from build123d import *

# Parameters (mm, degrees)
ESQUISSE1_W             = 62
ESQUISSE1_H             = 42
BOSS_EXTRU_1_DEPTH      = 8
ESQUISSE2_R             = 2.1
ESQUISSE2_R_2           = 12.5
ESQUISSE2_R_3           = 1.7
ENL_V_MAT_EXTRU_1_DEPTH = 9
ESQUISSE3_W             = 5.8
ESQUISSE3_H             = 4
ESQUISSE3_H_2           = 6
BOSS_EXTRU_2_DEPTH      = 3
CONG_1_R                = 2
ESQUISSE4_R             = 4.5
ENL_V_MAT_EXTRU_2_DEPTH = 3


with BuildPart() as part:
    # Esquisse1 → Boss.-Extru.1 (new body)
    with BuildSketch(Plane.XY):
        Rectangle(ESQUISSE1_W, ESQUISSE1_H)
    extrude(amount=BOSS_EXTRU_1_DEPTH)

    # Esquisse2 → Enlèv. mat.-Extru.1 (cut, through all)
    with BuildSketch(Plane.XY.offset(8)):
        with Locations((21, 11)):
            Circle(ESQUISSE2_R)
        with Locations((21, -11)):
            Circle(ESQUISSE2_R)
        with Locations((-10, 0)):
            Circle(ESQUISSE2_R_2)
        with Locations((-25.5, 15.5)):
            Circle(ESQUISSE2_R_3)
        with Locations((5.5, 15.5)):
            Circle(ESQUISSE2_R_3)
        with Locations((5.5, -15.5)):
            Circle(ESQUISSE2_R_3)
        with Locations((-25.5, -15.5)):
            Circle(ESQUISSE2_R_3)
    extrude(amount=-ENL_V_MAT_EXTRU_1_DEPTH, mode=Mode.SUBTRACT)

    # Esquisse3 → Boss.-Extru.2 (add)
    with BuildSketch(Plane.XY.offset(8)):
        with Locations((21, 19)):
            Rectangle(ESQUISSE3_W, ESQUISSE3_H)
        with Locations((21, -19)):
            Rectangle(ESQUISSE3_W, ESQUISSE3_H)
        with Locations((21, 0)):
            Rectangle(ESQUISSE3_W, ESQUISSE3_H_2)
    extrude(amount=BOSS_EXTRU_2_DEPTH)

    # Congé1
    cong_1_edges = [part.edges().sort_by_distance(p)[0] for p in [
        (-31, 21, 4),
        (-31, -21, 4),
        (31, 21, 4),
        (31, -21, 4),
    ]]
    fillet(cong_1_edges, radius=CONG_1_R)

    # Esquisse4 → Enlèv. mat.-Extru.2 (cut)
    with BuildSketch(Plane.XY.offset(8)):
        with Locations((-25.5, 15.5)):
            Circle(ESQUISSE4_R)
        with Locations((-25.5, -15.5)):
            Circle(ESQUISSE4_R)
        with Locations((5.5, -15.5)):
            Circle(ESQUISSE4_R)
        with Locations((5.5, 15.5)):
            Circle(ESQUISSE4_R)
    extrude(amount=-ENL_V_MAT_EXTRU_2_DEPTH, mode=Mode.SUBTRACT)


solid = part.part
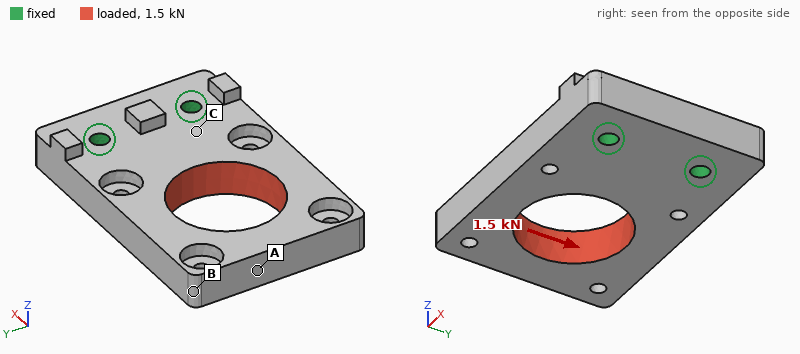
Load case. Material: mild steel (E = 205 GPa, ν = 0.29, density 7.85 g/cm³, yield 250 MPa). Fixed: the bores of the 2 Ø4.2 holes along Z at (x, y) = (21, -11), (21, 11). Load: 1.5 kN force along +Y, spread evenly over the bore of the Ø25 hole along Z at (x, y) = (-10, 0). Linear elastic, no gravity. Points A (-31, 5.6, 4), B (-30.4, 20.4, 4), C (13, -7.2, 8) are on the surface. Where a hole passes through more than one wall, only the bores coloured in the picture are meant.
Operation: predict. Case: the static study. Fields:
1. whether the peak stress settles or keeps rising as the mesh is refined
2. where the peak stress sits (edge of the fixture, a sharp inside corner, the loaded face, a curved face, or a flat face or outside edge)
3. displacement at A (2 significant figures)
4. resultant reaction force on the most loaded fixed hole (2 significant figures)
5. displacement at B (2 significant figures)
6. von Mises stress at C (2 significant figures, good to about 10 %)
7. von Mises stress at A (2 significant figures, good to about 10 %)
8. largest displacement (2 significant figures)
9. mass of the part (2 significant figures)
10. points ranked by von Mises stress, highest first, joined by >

keeps rising
a sharp inside corner
14 µm
2.0 kN
15 µm
16 MPa
10 MPa
16 µm
130 g
C > A > B
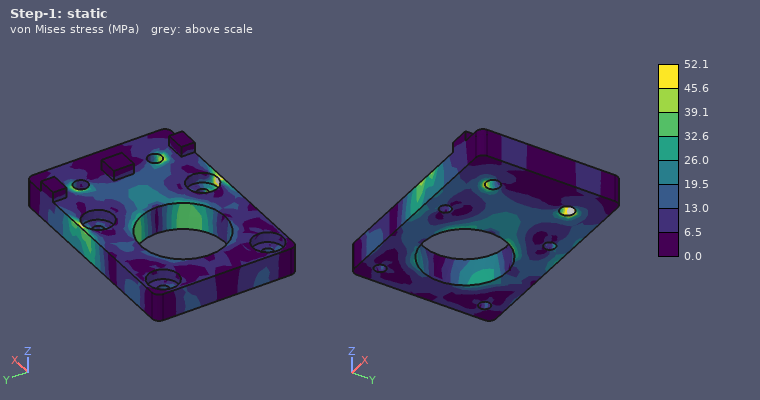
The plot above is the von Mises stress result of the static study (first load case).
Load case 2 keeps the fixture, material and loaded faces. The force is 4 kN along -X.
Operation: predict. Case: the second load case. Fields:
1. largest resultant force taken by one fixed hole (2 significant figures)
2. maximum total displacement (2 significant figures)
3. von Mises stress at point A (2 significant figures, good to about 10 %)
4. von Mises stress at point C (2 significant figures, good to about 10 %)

2.0 kN
11 µm
20 MPa
16 MPa
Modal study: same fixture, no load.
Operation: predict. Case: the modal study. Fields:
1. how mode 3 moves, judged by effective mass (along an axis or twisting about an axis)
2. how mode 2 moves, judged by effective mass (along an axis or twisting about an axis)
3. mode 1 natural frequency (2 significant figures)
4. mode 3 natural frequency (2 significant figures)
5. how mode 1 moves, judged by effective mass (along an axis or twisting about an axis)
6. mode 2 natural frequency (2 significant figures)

along Y
twisting about X
2300 Hz
6600 Hz
along Z
5200 Hz
